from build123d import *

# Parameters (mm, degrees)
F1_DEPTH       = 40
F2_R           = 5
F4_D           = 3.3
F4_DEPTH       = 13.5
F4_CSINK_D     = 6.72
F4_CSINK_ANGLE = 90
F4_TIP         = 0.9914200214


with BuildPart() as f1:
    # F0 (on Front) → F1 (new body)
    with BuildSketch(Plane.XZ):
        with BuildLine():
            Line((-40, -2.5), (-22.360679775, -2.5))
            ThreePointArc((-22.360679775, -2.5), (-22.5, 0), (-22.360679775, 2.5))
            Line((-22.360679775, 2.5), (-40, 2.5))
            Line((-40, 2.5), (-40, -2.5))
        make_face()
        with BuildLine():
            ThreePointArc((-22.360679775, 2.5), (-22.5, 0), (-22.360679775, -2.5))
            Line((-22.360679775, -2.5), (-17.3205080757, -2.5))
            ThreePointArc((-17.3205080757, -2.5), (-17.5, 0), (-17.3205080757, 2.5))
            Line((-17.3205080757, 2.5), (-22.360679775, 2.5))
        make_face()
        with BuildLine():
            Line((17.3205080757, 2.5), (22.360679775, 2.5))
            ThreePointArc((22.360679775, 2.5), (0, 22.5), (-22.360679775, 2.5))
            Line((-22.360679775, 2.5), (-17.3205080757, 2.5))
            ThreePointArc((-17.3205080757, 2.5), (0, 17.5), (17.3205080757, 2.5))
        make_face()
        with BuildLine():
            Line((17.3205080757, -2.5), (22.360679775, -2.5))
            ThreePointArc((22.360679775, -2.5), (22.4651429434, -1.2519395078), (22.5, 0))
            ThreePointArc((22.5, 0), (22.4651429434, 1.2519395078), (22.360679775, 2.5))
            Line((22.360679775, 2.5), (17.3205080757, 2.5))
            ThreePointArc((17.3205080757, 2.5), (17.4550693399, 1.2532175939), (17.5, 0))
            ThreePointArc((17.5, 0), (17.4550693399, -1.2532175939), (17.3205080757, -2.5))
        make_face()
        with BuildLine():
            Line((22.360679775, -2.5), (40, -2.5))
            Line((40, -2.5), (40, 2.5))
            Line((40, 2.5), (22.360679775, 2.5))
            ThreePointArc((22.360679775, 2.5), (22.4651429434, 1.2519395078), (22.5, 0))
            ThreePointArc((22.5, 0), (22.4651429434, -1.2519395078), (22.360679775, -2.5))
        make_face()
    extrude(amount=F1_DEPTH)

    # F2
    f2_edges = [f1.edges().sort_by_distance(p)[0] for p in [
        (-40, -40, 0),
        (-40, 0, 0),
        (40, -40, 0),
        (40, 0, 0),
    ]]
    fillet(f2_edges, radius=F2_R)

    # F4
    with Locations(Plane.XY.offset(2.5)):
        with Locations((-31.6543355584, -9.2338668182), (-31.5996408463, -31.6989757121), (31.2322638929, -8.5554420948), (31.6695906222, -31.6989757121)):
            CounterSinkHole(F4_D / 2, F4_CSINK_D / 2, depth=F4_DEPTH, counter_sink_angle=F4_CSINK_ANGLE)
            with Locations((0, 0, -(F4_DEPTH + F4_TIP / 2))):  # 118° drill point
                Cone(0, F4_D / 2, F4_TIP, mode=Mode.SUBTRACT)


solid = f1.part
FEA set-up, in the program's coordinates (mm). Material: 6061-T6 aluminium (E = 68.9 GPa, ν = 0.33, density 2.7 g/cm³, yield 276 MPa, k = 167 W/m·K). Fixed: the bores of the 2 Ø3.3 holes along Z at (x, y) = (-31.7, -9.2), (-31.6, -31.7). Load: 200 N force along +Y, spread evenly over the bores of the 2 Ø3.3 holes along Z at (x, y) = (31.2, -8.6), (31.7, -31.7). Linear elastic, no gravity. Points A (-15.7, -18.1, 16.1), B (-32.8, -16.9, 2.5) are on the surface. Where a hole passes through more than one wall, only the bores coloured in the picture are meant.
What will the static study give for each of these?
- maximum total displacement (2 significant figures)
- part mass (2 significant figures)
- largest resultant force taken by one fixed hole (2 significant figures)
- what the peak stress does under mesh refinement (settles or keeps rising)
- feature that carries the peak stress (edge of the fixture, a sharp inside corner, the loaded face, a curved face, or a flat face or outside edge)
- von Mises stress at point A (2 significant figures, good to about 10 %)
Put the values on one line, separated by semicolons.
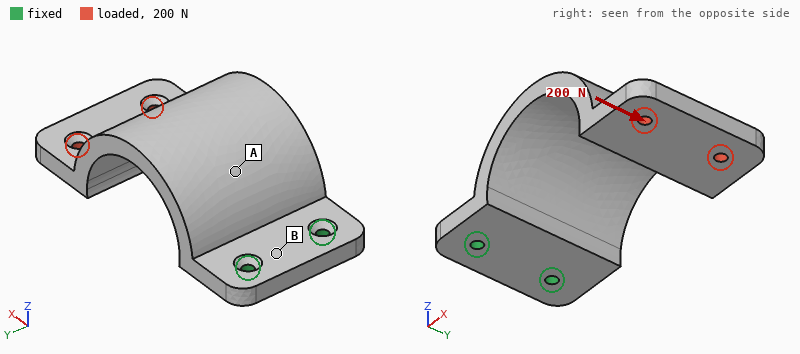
0.27 mm; 55 g; 530 N; keeps rising; edge of the fixture; 34 MPa
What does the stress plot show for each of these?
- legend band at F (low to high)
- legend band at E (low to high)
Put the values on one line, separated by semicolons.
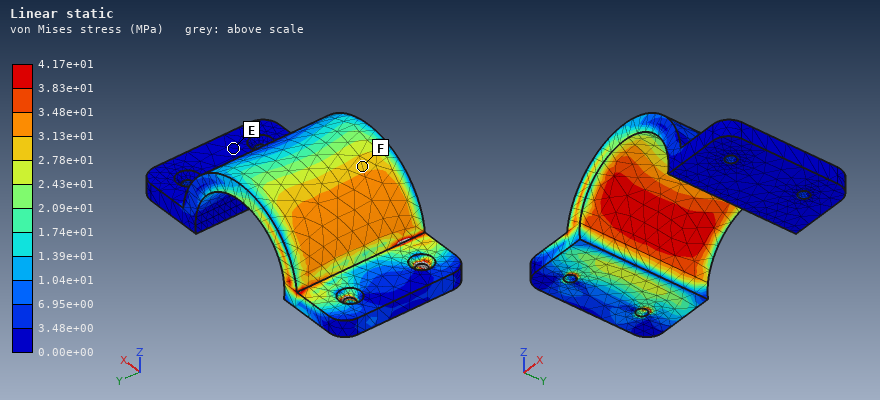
2.78e+01 to 3.13e+01 MPa; 0.00e+00 to 3.48e+00 MPa
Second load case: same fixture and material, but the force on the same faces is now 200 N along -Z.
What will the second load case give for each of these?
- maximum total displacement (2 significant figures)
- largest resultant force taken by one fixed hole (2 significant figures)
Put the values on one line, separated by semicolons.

1.0 mm; 100 N
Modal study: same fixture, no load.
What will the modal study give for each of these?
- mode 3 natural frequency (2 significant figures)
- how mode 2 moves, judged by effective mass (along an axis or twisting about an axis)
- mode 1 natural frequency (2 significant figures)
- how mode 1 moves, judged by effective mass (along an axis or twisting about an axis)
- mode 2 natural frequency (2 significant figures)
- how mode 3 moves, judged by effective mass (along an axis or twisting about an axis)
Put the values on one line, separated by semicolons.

1900 Hz; along Y; 580 Hz; along Z; 1200 Hz; along X
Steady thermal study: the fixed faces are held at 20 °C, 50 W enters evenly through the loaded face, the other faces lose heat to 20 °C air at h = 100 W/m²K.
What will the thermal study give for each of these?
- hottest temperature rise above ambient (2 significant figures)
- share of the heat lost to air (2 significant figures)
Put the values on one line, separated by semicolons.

77 K; 61 %
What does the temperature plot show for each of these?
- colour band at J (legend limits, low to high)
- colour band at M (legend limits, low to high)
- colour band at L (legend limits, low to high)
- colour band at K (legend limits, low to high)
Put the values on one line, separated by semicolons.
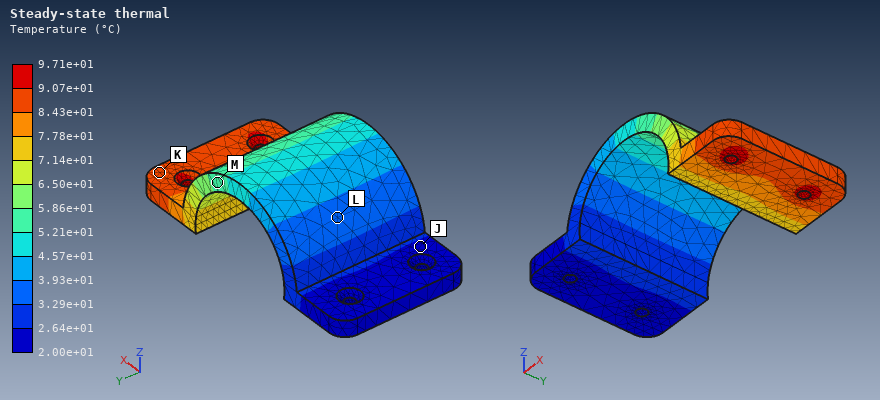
2.00e+01 to 2.64e+01 °C; 5.21e+01 to 5.86e+01 °C; 3.29e+01 to 3.93e+01 °C; 8.43e+01 to 9.07e+01 °C
